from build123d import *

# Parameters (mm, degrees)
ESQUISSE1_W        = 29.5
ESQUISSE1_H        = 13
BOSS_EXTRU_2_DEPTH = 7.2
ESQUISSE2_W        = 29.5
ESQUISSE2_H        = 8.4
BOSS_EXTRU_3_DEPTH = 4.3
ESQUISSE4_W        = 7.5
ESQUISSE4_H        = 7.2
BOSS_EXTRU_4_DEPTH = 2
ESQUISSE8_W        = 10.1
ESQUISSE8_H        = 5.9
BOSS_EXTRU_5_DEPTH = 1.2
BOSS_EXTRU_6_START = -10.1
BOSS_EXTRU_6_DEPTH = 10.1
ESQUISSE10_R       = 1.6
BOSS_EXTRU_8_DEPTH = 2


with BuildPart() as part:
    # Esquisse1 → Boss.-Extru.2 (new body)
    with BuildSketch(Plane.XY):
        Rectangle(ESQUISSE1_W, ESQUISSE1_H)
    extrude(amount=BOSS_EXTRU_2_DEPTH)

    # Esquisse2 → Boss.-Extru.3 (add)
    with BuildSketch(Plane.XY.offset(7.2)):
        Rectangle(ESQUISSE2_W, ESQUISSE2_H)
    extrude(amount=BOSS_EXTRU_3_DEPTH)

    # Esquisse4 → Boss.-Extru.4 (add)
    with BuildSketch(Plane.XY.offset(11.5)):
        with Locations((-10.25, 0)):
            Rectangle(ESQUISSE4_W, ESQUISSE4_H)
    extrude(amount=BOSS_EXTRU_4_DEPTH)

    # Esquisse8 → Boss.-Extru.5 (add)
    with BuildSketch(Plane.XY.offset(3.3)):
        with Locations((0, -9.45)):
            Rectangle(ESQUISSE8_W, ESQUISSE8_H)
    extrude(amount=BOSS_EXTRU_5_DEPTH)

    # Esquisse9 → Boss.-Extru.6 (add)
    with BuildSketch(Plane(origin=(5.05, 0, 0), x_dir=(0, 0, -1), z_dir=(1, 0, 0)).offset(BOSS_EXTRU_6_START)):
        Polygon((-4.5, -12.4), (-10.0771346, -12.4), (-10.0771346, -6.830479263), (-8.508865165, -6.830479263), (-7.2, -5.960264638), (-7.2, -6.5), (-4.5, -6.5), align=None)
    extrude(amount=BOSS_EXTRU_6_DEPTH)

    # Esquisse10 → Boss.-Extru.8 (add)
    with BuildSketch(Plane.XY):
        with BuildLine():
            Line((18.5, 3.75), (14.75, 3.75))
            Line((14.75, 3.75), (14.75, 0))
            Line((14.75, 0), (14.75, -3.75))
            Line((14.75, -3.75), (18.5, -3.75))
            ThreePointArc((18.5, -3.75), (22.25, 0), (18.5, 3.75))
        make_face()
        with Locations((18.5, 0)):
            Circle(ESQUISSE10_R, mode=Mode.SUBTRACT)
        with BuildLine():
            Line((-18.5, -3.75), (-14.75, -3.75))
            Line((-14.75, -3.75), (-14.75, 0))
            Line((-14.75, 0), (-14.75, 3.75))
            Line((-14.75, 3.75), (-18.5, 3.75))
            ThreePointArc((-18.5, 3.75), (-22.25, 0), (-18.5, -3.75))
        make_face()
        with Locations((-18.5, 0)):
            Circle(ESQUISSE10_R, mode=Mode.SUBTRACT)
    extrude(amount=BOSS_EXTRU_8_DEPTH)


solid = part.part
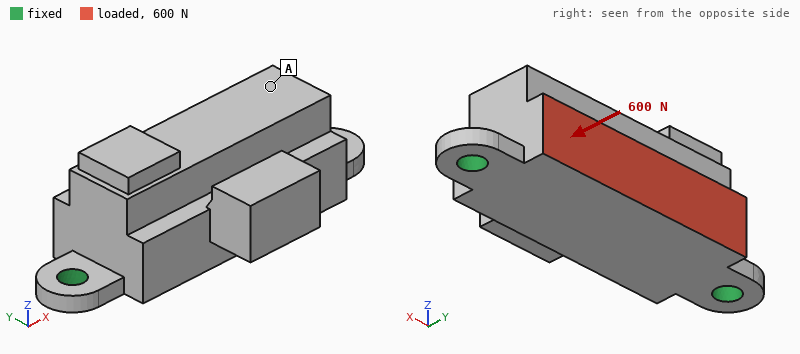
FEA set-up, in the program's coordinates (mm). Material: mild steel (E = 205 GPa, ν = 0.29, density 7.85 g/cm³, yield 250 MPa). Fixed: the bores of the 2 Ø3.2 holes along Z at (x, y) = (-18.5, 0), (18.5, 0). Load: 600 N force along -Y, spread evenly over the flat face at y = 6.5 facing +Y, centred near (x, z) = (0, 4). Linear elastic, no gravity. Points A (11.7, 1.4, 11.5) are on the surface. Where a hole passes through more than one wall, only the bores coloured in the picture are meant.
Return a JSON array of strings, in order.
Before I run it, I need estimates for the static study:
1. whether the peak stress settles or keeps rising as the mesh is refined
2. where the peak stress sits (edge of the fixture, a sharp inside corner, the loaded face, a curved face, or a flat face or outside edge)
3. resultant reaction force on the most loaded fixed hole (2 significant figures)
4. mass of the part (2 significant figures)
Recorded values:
["keeps rising", "edge of the fixture", "300 N", "35 g"]
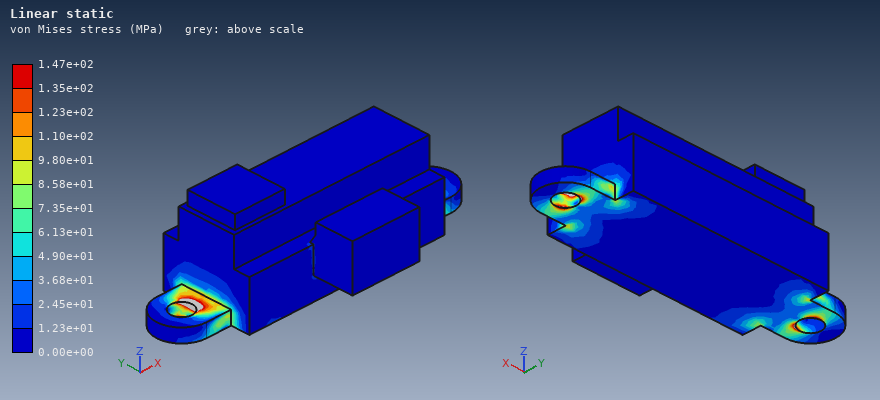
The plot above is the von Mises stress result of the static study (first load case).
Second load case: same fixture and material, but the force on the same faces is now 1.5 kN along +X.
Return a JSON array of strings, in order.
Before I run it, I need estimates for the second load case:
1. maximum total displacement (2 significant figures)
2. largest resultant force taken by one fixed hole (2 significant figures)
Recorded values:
["3.5 µm", "810 N"]
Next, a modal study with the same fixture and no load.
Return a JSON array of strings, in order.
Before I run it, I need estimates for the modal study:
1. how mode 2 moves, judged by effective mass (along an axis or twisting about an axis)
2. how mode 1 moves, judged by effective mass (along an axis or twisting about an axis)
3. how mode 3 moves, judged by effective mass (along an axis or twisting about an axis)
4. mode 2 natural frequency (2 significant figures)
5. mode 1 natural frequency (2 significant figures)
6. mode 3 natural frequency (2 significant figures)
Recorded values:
["along Z", "along Y", "along Y", "12 kHz", "4200 Hz", "19 kHz"]
